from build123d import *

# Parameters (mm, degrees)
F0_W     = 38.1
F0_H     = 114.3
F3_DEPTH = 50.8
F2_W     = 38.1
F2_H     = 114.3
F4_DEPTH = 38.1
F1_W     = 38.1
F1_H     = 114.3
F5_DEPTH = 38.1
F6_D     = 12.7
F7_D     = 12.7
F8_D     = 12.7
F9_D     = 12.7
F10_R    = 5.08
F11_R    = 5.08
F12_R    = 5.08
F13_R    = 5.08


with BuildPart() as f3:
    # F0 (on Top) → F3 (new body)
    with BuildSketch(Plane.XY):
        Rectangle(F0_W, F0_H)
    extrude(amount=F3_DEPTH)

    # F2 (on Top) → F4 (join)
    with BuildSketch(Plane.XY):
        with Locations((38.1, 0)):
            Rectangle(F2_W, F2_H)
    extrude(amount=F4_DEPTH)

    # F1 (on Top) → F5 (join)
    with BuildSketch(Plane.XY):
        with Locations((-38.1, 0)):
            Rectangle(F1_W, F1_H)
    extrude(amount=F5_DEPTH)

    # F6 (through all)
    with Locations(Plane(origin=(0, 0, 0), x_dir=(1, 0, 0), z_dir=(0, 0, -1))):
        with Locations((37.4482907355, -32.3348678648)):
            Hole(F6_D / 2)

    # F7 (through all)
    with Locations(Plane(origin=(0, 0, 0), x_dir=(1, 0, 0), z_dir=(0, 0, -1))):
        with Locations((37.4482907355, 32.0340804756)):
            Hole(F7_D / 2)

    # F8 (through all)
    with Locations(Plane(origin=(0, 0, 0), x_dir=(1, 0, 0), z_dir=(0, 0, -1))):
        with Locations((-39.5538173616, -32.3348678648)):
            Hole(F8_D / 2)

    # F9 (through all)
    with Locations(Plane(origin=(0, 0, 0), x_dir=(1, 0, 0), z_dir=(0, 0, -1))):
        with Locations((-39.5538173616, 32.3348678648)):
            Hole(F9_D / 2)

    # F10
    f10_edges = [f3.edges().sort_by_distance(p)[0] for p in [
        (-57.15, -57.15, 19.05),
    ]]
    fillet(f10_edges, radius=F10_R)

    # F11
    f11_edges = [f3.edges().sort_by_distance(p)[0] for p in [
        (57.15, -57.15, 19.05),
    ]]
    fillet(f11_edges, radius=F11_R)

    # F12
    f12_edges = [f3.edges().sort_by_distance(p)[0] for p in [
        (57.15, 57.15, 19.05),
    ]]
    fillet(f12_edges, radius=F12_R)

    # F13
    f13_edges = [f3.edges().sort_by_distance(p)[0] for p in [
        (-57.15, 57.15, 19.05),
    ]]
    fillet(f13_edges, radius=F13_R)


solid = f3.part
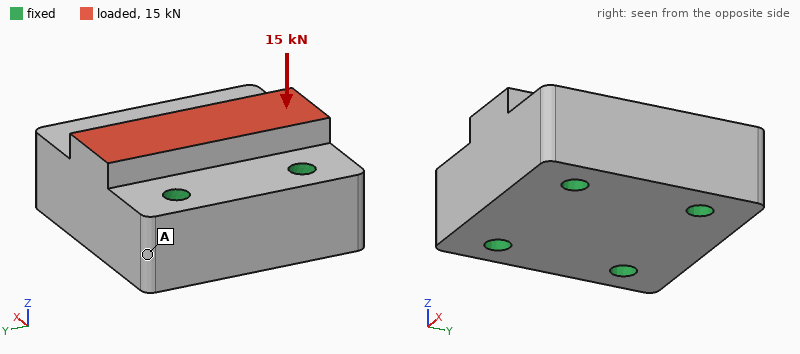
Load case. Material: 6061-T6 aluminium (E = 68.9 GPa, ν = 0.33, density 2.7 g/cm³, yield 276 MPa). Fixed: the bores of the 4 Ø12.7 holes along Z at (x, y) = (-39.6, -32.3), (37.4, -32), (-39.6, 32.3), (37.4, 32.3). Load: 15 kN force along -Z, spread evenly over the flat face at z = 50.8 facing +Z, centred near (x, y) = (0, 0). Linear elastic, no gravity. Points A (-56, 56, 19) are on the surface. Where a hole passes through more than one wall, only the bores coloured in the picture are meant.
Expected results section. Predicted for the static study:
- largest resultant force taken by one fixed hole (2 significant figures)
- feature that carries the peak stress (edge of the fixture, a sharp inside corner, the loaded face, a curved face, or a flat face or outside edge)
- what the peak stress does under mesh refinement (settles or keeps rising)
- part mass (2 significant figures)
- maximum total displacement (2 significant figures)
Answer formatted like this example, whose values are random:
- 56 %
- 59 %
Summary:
- 4.0 kN
- edge of the fixture
- keeps rising
- 1.4 kg
- 4.2 µm
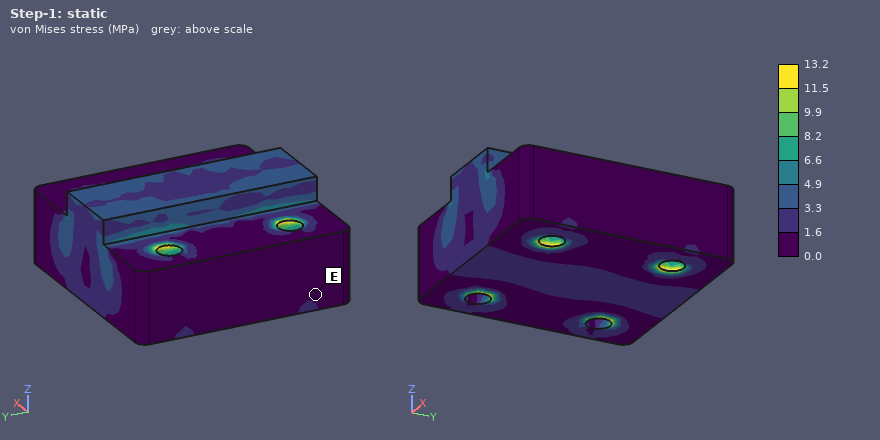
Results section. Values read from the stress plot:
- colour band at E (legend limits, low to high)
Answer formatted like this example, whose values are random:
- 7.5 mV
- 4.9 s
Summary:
- 0.0 to 1.6 MPa
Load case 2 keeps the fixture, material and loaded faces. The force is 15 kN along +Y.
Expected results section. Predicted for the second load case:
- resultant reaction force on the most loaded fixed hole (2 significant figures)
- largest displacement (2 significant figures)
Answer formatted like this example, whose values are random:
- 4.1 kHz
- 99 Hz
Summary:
- 4.8 kN
- 11 µm
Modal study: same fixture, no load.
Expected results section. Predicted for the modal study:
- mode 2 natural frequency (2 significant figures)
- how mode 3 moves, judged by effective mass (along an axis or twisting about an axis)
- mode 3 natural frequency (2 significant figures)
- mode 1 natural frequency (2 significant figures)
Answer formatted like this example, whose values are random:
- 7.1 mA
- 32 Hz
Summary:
- 14 kHz
- along Y
- 17 kHz
- 14 kHz
